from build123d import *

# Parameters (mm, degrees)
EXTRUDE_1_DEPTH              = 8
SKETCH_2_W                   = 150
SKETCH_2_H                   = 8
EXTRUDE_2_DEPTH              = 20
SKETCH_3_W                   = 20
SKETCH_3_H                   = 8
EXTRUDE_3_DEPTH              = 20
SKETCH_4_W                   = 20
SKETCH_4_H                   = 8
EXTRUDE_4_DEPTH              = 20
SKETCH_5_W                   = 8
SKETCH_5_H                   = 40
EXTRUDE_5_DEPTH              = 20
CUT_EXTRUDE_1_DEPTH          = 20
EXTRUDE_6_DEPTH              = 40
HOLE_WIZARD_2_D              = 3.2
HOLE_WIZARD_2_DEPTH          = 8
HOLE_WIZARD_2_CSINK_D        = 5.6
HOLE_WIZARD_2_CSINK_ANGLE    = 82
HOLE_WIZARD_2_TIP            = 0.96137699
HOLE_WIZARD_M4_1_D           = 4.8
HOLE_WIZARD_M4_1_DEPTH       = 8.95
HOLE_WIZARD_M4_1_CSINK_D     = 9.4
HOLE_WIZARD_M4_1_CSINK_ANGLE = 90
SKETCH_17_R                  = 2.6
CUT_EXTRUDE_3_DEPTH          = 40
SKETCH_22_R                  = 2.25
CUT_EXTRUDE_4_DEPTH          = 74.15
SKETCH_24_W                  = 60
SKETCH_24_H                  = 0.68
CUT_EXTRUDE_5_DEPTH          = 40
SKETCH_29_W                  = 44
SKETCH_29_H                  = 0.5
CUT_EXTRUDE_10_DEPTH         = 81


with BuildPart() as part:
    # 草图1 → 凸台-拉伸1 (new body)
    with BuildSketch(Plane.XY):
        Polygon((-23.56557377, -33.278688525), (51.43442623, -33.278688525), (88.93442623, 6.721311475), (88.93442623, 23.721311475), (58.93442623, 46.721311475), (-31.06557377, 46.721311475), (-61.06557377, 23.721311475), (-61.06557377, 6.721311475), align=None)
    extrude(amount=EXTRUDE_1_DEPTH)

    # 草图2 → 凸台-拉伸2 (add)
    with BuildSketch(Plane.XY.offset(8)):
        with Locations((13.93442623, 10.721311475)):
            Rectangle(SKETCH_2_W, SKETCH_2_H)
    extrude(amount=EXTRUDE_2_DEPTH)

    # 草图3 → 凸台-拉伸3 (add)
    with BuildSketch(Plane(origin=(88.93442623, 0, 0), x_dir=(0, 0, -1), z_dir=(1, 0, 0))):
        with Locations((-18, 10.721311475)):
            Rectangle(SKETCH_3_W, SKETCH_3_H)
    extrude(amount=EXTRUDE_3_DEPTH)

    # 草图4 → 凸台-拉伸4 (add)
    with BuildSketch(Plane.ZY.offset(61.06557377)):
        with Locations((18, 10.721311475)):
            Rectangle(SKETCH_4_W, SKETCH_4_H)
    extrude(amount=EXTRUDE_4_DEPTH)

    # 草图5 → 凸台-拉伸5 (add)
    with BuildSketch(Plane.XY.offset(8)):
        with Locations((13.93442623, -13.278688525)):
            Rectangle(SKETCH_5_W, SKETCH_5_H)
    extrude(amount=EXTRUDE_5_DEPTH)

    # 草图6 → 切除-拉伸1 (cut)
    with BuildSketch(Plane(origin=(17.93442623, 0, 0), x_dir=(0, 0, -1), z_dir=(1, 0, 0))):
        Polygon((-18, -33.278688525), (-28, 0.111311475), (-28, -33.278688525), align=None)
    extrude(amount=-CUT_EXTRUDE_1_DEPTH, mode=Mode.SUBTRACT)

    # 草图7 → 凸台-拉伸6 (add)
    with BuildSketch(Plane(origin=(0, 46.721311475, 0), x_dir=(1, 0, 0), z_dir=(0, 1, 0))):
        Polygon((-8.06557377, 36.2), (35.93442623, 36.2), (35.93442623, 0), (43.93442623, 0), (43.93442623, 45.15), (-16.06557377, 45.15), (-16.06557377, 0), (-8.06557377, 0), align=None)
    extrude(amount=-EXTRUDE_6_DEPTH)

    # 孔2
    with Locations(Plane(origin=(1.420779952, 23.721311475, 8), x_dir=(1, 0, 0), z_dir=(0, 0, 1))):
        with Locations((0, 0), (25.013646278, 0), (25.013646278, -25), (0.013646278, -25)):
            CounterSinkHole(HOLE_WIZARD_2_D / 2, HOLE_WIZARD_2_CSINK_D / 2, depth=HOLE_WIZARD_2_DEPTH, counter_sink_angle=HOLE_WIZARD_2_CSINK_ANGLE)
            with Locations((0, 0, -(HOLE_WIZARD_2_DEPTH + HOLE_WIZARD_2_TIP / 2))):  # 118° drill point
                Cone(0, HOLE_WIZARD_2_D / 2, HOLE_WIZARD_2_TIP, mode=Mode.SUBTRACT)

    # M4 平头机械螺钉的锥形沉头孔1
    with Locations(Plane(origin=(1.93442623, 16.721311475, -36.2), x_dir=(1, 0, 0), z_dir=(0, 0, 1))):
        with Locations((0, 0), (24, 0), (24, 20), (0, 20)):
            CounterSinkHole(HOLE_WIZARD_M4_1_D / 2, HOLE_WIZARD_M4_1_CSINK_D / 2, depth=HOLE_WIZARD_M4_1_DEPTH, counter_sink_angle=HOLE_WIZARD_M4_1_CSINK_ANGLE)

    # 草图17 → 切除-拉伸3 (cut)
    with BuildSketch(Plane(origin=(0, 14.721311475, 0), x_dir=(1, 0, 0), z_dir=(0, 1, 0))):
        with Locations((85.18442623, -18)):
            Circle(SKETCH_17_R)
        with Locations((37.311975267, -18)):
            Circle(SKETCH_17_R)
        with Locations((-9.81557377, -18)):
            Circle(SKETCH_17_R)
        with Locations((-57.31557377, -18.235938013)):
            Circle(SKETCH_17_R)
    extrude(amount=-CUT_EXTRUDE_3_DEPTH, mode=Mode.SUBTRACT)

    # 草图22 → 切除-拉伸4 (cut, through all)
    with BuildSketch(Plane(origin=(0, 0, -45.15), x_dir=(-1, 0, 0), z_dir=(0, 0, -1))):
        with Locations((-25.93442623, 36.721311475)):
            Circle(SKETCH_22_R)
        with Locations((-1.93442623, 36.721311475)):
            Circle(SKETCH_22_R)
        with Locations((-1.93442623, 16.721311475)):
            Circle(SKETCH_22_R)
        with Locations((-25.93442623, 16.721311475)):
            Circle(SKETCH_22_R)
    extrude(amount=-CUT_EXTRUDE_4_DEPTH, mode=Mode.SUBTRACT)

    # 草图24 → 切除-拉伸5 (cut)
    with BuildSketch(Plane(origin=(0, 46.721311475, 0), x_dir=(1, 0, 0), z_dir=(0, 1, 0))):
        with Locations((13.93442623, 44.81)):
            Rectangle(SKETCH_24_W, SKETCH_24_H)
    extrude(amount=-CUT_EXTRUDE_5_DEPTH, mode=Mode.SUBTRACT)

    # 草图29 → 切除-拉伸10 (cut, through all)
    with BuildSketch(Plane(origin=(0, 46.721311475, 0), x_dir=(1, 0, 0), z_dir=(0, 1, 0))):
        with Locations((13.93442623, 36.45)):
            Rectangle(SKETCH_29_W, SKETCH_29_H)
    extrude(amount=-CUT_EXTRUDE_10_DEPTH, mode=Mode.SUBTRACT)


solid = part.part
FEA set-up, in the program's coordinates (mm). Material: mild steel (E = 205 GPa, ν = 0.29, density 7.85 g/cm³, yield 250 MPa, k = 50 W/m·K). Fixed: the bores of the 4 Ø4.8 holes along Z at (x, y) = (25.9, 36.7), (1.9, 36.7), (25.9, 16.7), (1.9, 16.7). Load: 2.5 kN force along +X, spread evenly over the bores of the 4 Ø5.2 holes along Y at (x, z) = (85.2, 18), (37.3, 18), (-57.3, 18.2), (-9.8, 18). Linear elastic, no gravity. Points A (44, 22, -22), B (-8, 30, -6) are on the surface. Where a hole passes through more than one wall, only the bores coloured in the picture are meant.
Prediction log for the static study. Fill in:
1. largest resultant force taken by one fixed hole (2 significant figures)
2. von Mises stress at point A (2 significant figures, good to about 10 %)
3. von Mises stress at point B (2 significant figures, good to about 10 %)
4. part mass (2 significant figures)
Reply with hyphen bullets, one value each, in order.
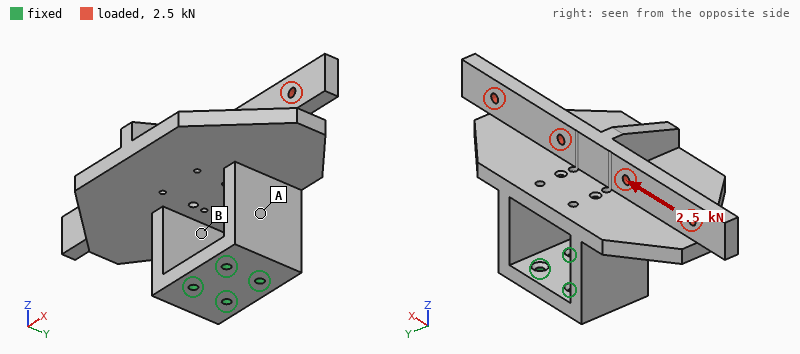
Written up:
- 2.0 kN
- 12 MPa
- 46 MPa
- 1.2 kg
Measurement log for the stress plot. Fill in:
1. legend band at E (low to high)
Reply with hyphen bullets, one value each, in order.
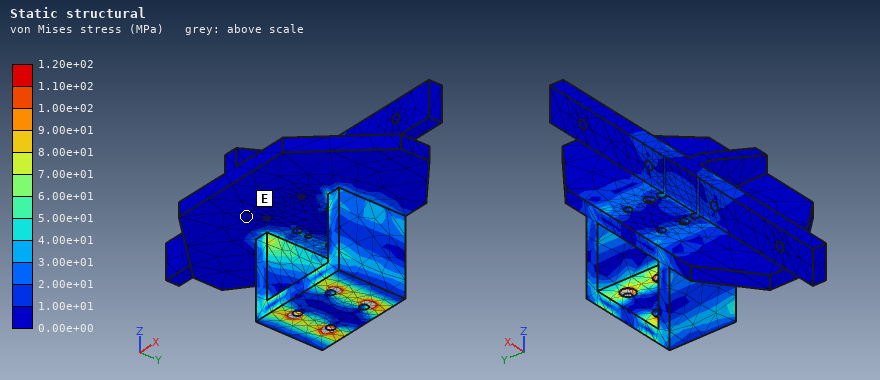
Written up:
- 0.00e+00 to 1.00e+01 MPa
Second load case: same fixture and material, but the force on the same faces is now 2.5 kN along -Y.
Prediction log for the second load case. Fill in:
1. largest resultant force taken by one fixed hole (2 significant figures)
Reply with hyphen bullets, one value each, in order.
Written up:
- 3.1 kN
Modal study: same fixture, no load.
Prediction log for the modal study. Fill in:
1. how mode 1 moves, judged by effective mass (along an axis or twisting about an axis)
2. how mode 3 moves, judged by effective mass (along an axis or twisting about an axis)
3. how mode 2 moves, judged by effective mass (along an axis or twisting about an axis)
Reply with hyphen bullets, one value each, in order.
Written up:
- along X
- twisting about Z
- along Y
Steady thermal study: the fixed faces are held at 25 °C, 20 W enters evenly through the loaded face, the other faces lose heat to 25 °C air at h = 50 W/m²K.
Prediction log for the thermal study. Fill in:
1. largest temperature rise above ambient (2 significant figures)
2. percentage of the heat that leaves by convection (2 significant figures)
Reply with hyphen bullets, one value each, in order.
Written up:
- 17 K
- 82 %
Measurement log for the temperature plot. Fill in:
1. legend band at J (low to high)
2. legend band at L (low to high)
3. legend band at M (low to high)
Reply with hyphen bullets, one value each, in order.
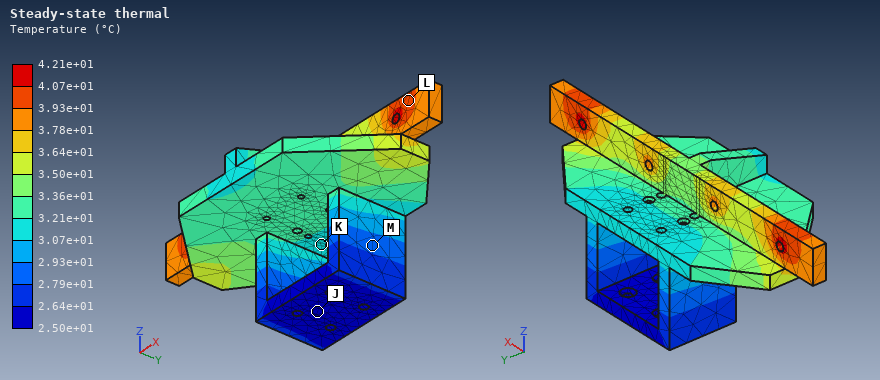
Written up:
- 2.50e+01 to 2.64e+01 °C
- 3.93e+01 to 4.07e+01 °C
- 2.79e+01 to 2.93e+01 °C
